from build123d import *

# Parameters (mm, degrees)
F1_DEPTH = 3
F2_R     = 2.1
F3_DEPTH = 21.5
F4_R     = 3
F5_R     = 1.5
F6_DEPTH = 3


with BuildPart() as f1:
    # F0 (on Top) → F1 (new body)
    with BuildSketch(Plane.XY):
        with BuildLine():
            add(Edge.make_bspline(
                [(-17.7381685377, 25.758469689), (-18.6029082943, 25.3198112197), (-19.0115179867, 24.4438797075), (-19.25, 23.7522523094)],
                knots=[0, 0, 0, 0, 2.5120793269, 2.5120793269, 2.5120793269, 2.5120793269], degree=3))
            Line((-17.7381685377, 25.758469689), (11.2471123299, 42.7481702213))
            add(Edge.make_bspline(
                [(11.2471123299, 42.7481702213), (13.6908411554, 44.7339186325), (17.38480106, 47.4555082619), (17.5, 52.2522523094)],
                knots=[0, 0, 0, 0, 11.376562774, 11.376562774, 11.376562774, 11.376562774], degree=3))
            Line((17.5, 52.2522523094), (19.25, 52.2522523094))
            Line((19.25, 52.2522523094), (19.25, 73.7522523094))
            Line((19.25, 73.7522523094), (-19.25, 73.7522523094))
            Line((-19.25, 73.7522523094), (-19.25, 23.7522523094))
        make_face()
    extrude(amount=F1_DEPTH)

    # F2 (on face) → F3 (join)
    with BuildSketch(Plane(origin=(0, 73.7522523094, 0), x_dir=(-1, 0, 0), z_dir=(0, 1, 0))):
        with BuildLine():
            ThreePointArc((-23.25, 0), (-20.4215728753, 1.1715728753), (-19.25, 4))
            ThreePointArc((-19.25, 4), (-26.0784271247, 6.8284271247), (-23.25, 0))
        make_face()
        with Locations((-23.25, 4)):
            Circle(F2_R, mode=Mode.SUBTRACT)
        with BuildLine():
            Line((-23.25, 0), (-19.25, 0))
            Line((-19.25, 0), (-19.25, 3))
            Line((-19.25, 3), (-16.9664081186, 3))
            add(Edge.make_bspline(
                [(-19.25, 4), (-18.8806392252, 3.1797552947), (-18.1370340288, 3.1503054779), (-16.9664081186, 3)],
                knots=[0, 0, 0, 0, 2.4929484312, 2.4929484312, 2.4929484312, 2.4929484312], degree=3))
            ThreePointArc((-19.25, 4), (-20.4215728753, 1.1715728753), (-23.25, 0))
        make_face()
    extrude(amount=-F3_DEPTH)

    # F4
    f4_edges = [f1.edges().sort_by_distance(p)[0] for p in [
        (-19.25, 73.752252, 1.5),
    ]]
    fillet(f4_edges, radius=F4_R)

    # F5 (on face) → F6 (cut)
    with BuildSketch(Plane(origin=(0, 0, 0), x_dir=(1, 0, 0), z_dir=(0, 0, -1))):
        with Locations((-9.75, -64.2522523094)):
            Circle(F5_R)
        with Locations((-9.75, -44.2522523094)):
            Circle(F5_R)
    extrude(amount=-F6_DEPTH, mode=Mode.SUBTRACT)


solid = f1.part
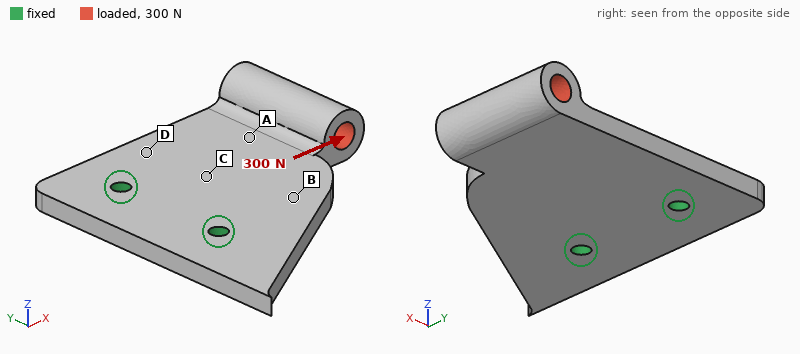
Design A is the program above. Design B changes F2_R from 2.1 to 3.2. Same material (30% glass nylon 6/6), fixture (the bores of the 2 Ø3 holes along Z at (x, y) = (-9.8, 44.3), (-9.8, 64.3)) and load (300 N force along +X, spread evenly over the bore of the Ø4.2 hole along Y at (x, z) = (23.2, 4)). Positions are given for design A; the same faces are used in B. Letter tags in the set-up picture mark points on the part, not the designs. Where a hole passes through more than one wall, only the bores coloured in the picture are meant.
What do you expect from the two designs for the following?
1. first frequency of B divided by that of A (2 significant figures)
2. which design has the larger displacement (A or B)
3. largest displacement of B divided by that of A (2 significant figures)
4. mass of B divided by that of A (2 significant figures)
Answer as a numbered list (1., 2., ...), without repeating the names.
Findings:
1. 1.2
2. B
3. 1.2
4. 0.92
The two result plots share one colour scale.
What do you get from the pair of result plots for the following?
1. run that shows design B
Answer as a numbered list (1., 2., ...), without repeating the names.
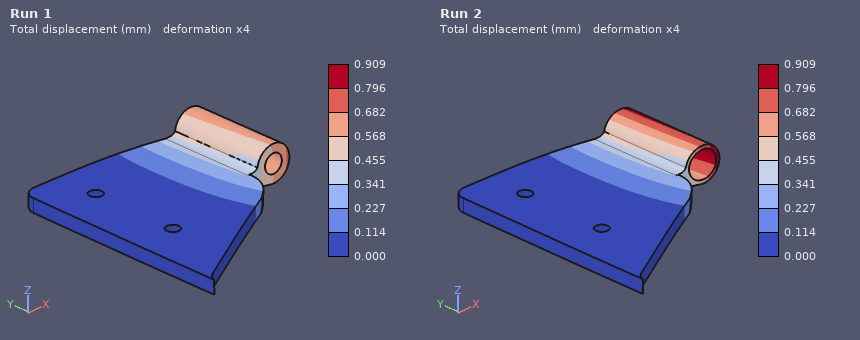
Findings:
1. Run 2
